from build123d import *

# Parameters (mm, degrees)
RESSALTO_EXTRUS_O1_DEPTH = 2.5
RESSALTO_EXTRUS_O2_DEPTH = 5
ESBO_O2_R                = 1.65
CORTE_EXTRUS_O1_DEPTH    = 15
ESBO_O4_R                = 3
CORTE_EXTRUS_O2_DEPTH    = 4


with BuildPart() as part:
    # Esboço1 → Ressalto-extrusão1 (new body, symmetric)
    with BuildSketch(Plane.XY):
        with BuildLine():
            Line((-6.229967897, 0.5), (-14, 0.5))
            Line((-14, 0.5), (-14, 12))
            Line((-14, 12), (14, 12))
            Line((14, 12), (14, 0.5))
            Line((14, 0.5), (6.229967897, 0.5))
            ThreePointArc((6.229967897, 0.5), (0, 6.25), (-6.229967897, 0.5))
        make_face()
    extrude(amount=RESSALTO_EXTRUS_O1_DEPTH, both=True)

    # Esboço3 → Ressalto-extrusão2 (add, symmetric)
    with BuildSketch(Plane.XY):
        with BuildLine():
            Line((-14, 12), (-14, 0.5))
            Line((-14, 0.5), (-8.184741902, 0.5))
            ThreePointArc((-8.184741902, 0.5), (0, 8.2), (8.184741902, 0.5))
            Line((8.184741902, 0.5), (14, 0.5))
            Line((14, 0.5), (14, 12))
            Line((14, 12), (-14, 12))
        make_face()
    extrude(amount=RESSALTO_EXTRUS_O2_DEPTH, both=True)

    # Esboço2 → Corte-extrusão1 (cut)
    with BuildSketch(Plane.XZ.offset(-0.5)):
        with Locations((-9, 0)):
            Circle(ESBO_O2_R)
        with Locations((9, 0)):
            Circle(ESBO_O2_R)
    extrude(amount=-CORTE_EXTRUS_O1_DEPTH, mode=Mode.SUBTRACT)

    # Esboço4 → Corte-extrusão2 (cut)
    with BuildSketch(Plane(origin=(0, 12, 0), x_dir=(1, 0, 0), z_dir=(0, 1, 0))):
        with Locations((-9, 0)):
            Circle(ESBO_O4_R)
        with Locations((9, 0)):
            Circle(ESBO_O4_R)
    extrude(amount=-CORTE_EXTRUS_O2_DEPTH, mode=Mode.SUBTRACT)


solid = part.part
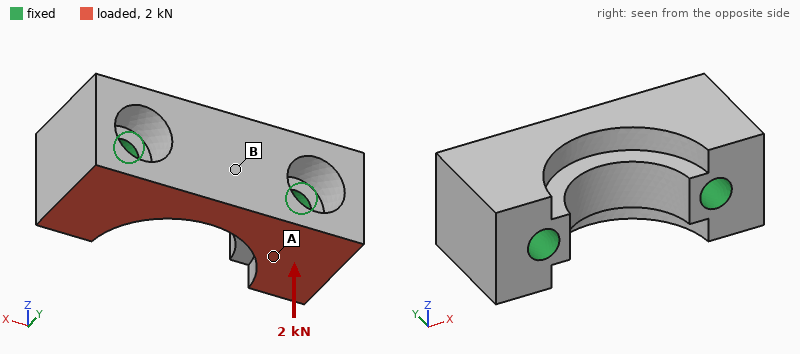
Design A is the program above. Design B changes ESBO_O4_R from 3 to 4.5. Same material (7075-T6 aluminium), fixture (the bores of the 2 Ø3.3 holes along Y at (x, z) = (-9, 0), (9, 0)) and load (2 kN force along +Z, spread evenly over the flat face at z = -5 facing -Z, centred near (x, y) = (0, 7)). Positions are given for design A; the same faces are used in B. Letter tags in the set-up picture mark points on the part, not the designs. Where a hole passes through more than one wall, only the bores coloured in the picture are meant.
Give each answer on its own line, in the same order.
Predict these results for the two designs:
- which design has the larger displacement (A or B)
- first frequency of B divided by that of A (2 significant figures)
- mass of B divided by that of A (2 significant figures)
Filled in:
B
0.88
0.87
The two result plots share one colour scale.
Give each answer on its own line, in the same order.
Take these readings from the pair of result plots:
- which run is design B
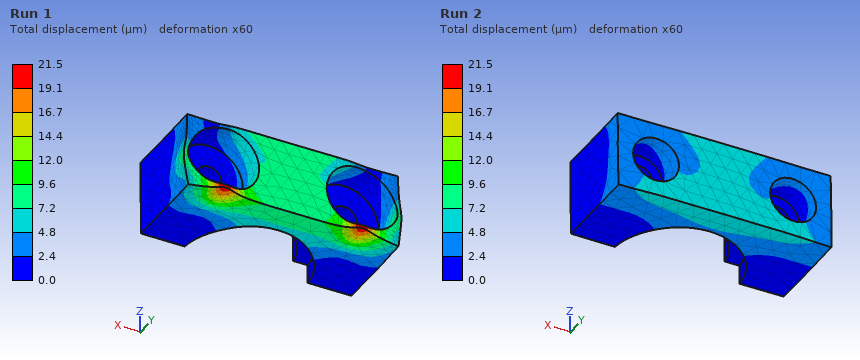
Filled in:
Run 1
